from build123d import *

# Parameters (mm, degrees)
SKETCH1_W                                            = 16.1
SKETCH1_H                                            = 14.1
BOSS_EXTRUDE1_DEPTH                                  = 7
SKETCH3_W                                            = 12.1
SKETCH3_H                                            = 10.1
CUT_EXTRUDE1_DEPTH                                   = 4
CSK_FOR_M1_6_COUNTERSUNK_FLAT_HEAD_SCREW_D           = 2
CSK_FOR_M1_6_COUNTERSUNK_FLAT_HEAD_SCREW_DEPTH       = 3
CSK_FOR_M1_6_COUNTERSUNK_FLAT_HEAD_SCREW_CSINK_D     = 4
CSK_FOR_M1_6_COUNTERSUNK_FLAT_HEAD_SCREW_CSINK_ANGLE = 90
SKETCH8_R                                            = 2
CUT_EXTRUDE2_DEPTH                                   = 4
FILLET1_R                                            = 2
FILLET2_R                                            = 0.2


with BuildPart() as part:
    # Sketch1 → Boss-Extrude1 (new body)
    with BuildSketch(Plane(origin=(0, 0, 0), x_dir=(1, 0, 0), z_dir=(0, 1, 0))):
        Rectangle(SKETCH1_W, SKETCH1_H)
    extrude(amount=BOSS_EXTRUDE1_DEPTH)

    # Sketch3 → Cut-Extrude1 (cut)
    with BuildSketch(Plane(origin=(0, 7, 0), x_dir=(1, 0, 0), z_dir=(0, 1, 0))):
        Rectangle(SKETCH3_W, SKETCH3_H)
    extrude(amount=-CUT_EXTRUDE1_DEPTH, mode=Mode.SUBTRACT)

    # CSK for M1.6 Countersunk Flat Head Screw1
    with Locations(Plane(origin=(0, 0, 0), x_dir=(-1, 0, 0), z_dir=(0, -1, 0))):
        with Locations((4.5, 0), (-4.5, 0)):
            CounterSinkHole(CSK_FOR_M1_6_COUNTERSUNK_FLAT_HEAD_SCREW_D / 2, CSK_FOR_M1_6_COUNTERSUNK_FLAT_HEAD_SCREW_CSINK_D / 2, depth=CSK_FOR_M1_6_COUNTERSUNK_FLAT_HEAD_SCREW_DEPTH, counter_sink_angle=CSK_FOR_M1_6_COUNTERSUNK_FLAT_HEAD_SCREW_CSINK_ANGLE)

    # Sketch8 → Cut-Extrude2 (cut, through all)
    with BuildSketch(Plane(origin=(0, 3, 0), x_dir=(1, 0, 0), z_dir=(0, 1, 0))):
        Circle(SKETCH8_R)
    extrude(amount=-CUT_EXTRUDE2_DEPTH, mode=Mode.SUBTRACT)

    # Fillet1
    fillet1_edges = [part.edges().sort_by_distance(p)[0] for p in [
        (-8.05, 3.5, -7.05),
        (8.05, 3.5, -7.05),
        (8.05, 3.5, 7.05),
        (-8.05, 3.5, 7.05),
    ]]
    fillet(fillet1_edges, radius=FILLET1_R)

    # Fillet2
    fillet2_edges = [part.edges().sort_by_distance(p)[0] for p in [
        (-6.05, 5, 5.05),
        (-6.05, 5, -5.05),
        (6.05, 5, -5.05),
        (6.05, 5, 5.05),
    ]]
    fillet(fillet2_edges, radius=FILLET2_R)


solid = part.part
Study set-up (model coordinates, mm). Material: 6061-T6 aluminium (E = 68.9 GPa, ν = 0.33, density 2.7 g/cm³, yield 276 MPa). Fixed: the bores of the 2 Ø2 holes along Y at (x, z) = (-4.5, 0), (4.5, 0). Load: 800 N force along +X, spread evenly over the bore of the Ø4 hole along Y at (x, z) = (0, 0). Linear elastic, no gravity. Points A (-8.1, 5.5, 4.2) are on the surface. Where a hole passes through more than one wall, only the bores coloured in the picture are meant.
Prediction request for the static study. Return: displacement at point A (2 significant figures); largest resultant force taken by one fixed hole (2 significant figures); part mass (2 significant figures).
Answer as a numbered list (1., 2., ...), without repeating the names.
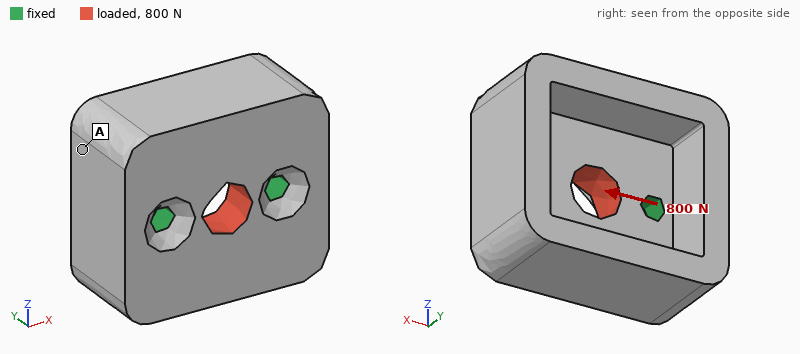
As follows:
1. 0.58 µm
2. 400 N
3. 2.7 g
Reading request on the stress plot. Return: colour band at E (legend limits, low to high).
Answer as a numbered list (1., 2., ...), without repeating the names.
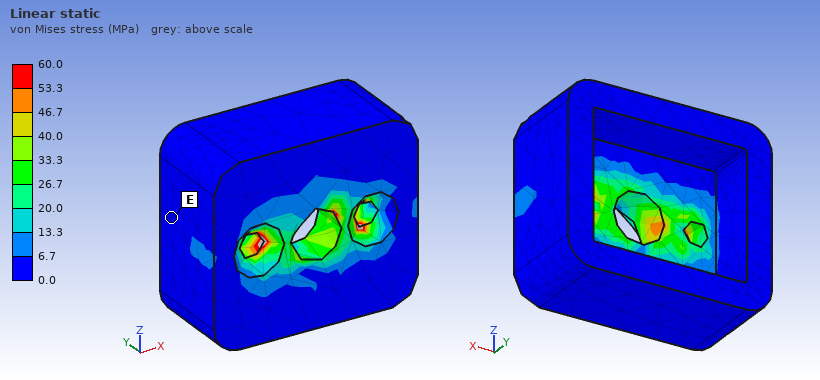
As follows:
1. 0.0 to 6.7 MPa
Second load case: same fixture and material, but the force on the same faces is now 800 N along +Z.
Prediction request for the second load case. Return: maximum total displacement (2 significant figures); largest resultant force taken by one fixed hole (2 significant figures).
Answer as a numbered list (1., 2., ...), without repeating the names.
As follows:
1. 2.6 µm
2. 400 N
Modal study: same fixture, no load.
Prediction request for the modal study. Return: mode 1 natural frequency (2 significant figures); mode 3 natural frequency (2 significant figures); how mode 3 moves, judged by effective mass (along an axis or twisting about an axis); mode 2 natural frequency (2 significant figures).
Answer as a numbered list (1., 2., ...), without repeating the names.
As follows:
1. 20 kHz
2. 41 kHz
3. along Y
4. 33 kHz
